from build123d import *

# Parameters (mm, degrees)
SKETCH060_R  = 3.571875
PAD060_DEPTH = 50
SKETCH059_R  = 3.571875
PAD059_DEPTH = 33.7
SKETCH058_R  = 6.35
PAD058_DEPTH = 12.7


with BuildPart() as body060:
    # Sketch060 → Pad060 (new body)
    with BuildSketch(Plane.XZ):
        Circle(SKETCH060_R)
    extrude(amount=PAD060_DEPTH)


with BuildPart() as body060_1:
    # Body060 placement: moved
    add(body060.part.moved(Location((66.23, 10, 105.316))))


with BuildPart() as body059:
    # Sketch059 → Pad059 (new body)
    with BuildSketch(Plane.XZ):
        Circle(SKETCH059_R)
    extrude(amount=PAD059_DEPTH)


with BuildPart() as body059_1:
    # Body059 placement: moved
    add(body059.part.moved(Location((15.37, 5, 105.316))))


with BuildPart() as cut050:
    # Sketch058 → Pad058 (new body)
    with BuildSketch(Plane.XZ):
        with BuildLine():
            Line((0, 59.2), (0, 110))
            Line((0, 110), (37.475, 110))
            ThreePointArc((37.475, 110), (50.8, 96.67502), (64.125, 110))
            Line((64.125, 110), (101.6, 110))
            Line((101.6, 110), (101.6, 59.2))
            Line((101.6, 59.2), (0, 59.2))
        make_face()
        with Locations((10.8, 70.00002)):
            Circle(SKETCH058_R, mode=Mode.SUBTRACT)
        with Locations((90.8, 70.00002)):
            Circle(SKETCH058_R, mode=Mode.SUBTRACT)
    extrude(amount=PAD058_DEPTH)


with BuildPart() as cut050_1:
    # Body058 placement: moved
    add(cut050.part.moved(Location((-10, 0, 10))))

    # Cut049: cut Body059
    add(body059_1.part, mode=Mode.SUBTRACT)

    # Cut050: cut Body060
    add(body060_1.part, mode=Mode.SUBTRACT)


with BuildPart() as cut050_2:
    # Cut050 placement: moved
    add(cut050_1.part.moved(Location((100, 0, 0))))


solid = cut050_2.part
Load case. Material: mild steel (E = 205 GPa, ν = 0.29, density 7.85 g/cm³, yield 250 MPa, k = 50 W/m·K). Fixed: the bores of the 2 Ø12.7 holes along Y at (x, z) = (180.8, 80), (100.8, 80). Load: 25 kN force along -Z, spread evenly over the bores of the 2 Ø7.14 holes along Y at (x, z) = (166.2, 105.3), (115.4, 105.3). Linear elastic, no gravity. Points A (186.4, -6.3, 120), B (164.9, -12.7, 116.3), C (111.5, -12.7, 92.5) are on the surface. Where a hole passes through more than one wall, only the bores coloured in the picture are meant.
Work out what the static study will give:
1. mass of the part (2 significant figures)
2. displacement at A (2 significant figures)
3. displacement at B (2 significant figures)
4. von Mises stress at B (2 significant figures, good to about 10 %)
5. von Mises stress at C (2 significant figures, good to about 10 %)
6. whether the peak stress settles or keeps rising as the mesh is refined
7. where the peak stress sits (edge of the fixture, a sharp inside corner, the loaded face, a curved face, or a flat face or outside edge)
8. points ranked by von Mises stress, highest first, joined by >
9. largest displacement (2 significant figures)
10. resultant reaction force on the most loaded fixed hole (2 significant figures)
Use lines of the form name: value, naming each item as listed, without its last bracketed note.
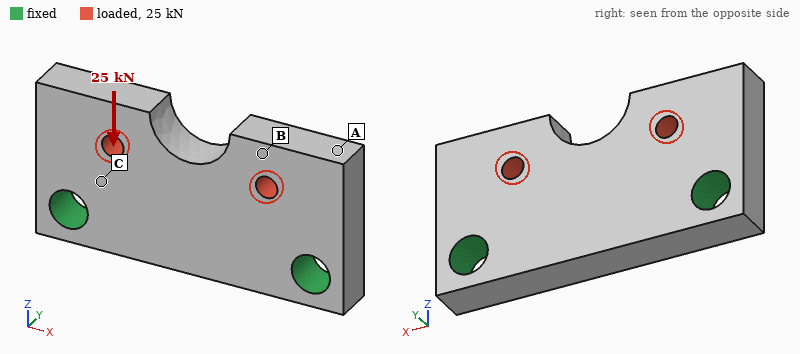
mass of the part: 450 g
displacement at A: 5.8 µm
displacement at B: 8.4 µm
von Mises stress at B: 23 MPa
von Mises stress at C: 49 MPa
whether the peak stress settles or keeps rising as the mesh is refined: keeps rising
where the peak stress sits: edge of the fixture
points ranked by von Mises stress, highest first, joined by >: C > B > A
largest displacement: 9.0 µm
resultant reaction force on the most loaded fixed hole: 13 kN
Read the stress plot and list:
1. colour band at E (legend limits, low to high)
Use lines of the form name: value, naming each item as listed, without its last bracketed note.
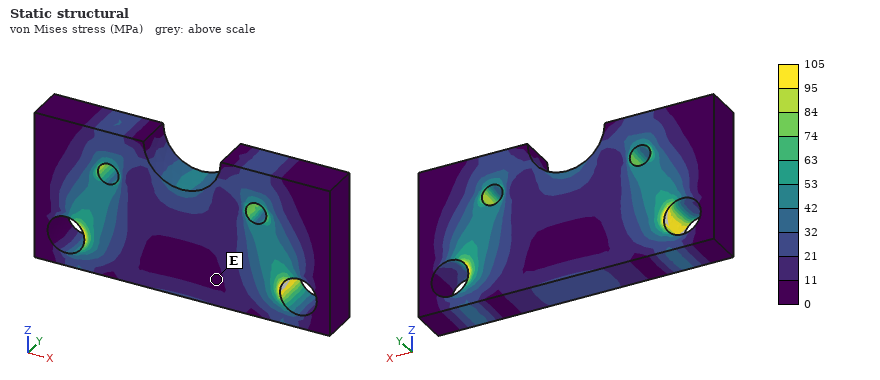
colour band at E: 0 to 11 MPa
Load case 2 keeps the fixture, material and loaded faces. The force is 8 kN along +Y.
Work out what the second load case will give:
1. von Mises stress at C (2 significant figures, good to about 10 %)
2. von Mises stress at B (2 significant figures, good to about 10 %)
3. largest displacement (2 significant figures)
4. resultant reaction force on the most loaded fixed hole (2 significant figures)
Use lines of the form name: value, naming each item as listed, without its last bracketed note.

von Mises stress at C: 49 MPa
von Mises stress at B: 25 MPa
largest displacement: 41 µm
resultant reaction force on the most loaded fixed hole: 4.0 kN
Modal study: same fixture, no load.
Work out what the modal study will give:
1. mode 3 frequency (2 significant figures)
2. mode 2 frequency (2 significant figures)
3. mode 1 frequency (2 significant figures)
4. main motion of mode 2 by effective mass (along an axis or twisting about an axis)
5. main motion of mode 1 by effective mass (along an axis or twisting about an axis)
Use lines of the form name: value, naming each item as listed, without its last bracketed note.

mode 3 frequency: 10 kHz
mode 2 frequency: 8300 Hz
mode 1 frequency: 5900 Hz
main motion of mode 2 by effective mass: twisting about Z
main motion of mode 1 by effective mass: along Y
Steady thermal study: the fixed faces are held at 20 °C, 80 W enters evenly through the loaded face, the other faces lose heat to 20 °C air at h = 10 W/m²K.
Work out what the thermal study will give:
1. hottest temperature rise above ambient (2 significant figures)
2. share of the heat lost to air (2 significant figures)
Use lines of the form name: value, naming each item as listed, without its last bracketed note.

hottest temperature rise above ambient: 52 K
share of the heat lost to air: 3.9 %
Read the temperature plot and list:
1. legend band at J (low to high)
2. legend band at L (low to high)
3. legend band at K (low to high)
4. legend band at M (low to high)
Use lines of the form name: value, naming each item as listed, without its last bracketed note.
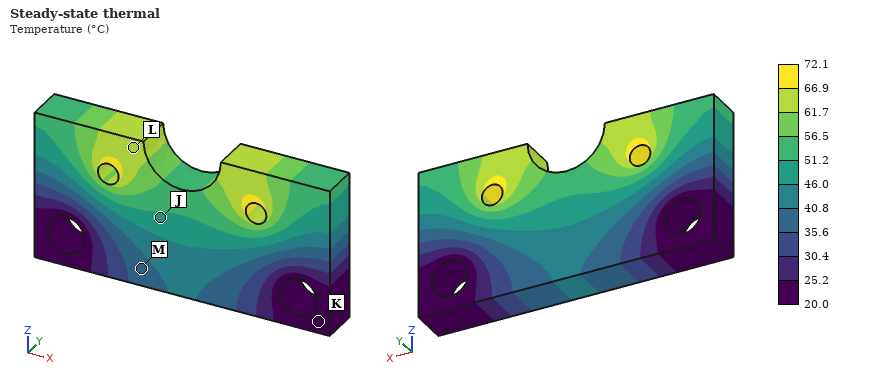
legend band at J: 46.0 to 51.2 °C
legend band at L: 61.7 to 66.9 °C
legend band at K: 20.0 to 25.2 °C
legend band at M: 35.6 to 40.8 °C
